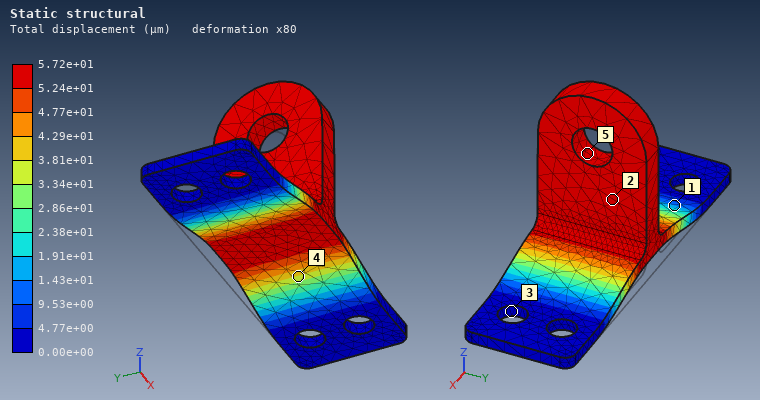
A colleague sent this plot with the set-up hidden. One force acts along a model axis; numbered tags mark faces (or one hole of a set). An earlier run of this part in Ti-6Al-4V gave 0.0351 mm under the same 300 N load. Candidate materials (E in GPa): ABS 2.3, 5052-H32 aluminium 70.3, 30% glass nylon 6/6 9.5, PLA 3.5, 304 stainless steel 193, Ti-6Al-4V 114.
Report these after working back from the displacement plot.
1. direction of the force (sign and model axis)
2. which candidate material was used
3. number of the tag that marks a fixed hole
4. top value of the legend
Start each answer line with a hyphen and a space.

- +Z
- 5052-H32 aluminium
- 3
- 5.72e+01 µm
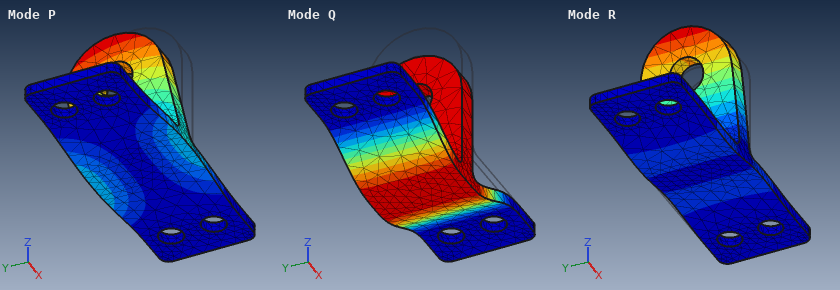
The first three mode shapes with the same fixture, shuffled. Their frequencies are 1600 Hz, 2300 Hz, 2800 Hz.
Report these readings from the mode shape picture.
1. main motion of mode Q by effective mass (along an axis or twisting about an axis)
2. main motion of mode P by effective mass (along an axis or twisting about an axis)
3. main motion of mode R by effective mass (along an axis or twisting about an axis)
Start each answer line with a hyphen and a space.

- along Z
- along Y
- along X
